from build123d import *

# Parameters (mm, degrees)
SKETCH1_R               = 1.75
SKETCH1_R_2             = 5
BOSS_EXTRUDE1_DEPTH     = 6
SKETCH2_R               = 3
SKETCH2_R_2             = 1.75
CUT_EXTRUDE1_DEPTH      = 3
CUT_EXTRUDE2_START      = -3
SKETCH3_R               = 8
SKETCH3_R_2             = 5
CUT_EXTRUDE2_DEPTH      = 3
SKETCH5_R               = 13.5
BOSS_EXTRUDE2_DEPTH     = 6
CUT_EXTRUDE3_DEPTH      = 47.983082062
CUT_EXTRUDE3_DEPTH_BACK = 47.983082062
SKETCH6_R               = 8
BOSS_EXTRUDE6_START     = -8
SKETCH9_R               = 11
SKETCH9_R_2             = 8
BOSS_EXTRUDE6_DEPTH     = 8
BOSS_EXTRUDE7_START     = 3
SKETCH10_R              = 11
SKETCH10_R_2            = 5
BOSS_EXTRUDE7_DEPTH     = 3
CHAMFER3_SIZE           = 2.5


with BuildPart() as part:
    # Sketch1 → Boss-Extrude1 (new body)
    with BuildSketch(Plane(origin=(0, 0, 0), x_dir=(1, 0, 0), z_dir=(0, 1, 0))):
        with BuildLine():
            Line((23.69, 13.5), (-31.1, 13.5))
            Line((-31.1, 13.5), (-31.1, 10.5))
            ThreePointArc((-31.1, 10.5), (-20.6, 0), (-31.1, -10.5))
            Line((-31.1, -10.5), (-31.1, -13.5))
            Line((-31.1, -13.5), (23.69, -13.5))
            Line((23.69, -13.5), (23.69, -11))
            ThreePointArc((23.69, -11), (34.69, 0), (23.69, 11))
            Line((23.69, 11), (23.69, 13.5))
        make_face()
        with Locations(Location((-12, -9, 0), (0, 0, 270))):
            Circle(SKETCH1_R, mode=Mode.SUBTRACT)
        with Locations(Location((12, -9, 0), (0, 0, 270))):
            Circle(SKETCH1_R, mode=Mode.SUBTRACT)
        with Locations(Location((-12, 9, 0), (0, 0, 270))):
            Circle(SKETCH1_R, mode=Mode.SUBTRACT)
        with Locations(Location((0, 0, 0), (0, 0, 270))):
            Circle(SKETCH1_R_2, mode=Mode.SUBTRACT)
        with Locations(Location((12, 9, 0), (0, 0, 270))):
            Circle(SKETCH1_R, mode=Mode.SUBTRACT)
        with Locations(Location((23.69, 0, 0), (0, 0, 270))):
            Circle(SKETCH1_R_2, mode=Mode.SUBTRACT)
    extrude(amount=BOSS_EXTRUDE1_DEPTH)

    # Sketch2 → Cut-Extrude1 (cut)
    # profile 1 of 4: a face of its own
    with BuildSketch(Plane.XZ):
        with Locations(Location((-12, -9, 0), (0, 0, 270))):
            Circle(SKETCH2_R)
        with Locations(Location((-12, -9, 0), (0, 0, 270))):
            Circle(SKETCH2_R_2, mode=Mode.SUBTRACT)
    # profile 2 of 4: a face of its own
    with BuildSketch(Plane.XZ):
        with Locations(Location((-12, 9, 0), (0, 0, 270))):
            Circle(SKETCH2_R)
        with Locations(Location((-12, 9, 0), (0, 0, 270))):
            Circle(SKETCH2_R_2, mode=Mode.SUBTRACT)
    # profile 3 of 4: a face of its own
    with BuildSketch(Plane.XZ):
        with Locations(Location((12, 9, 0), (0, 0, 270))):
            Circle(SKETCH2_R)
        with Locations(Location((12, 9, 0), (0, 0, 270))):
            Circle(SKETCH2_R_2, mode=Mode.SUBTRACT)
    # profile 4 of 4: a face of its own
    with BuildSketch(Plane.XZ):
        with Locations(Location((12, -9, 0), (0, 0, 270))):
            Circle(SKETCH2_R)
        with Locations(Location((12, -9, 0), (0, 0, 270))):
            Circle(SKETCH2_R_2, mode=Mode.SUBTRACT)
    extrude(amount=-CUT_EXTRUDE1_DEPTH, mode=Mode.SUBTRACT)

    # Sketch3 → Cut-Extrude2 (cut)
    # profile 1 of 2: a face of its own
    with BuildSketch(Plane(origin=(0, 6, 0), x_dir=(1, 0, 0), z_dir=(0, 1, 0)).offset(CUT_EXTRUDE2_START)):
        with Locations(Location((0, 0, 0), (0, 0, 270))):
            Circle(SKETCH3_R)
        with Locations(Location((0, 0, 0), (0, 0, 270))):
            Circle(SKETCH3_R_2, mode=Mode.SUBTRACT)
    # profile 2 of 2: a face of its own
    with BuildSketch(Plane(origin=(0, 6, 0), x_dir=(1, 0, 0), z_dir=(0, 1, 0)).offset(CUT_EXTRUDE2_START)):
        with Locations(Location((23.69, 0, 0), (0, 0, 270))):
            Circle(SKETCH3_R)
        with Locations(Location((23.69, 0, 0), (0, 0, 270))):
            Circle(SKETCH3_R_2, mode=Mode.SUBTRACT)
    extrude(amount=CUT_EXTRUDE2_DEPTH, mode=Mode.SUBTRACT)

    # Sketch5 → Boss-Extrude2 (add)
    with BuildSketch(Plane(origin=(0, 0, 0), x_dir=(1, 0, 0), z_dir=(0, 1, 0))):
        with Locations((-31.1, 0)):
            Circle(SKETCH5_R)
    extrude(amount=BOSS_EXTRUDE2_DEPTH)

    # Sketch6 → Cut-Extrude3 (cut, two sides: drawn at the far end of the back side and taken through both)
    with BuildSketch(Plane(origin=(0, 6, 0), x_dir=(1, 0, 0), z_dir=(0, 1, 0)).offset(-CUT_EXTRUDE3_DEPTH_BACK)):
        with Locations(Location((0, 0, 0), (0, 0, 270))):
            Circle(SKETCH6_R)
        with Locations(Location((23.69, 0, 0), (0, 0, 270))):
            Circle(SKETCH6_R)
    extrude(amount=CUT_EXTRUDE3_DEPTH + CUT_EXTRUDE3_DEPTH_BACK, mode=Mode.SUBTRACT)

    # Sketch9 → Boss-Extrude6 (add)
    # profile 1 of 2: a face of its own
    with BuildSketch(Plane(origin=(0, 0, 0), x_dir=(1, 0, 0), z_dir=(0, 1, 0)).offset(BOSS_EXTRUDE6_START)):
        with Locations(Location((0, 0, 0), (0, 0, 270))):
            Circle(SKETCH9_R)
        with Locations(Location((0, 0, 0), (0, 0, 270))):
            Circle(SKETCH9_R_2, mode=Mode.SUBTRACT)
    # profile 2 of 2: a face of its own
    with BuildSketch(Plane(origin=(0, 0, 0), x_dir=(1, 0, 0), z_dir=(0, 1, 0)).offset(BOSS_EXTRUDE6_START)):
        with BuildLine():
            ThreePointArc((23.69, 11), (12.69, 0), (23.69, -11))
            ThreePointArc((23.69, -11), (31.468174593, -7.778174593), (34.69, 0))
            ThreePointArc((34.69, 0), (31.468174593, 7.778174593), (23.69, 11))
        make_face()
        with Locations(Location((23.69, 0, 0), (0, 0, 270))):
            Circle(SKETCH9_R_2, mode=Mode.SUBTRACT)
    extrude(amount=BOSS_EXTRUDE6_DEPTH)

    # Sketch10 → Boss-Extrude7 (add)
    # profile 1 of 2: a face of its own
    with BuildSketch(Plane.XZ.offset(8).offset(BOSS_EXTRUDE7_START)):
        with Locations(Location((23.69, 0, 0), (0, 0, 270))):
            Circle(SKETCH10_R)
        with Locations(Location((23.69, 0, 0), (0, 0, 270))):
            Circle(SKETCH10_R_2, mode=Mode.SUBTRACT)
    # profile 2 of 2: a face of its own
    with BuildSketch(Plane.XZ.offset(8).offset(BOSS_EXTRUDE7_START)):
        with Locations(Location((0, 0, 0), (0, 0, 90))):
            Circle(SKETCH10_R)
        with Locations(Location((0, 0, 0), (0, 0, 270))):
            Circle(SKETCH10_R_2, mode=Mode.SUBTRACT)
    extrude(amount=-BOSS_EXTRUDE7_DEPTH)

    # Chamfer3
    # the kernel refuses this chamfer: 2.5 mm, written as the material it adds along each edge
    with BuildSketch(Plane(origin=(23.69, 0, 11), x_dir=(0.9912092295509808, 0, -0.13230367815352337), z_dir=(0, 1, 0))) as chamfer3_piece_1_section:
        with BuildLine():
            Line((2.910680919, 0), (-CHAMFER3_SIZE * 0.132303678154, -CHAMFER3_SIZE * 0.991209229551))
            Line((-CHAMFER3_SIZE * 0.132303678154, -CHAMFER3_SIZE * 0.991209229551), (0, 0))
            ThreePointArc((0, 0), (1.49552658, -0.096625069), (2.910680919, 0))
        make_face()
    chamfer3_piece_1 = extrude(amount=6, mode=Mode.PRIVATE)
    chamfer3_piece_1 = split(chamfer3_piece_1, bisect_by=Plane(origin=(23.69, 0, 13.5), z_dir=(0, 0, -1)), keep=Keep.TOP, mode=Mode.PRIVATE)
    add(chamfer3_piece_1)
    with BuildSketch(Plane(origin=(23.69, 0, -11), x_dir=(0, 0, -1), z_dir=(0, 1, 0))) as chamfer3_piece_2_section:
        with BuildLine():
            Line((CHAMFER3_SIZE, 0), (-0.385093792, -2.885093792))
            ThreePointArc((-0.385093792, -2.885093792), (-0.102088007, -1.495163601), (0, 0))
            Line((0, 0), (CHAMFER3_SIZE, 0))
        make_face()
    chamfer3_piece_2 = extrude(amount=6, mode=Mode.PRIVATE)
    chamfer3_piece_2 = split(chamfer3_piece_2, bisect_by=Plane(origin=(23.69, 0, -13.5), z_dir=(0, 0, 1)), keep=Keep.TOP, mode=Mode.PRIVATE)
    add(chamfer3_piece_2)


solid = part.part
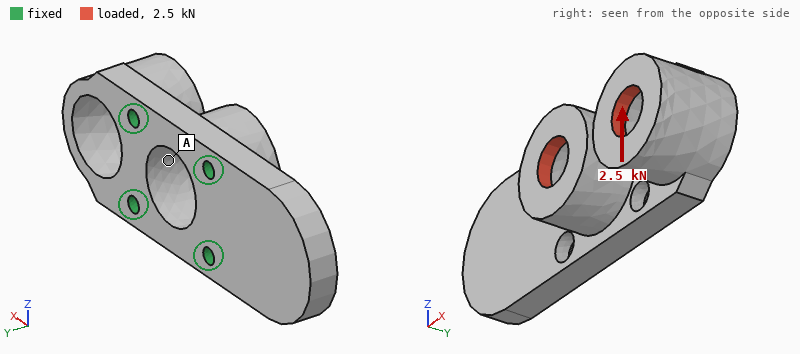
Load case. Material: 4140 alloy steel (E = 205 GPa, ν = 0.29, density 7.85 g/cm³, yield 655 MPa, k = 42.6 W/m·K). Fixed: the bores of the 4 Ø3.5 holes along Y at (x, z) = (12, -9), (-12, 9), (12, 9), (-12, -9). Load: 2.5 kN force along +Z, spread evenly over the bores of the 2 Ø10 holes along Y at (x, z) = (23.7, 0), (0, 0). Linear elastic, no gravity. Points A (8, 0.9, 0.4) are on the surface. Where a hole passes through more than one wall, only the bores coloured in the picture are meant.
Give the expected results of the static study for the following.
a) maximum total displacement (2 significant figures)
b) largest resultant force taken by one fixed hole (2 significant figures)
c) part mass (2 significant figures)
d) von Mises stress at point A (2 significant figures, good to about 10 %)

12 µm
1.7 kN
110 g
15 MPa
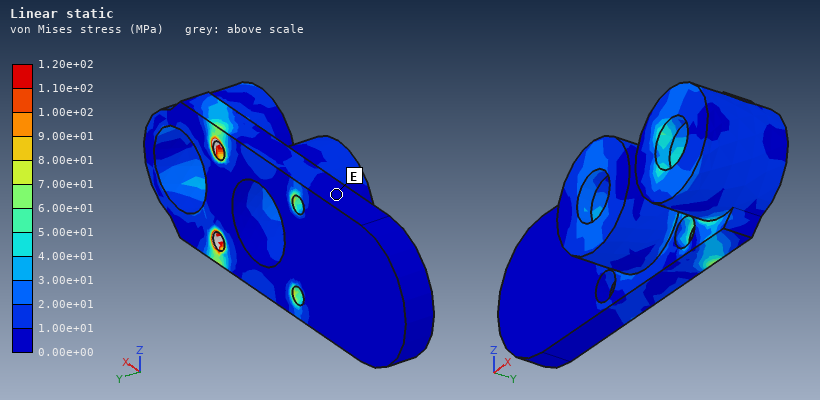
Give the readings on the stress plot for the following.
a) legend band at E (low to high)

0.00e+00 to 1.00e+01 MPa
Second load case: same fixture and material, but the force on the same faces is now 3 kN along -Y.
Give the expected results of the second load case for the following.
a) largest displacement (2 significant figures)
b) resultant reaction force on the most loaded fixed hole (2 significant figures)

47 µm
1.3 kN
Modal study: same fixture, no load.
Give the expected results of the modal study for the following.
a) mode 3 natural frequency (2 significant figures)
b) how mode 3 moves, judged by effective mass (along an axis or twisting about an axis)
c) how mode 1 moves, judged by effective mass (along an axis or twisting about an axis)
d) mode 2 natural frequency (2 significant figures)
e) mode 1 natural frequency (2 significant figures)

13 kHz
along Z
along Y
5800 Hz
4200 Hz
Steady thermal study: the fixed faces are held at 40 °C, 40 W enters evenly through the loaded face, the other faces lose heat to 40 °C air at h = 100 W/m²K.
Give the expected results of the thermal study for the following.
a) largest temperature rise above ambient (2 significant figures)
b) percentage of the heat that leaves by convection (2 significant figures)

62 K
38 %
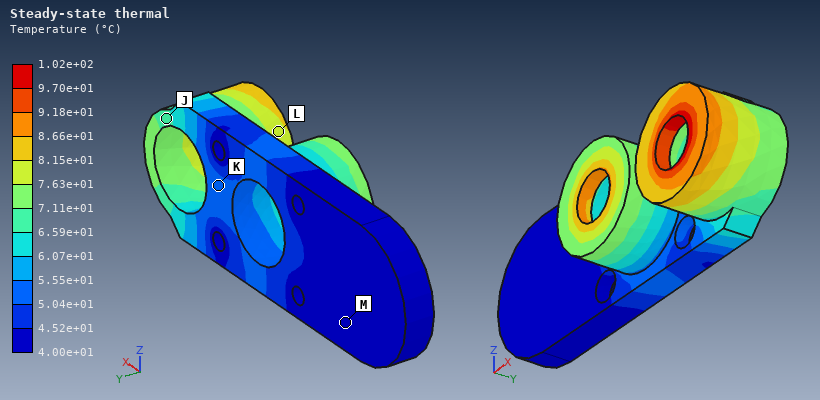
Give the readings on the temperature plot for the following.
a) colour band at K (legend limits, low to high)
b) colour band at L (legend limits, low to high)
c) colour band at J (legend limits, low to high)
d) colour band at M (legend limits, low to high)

5.04e+01 to 5.55e+01 °C
7.63e+01 to 8.15e+01 °C
6.59e+01 to 7.11e+01 °C
4.00e+01 to 4.52e+01 °C
